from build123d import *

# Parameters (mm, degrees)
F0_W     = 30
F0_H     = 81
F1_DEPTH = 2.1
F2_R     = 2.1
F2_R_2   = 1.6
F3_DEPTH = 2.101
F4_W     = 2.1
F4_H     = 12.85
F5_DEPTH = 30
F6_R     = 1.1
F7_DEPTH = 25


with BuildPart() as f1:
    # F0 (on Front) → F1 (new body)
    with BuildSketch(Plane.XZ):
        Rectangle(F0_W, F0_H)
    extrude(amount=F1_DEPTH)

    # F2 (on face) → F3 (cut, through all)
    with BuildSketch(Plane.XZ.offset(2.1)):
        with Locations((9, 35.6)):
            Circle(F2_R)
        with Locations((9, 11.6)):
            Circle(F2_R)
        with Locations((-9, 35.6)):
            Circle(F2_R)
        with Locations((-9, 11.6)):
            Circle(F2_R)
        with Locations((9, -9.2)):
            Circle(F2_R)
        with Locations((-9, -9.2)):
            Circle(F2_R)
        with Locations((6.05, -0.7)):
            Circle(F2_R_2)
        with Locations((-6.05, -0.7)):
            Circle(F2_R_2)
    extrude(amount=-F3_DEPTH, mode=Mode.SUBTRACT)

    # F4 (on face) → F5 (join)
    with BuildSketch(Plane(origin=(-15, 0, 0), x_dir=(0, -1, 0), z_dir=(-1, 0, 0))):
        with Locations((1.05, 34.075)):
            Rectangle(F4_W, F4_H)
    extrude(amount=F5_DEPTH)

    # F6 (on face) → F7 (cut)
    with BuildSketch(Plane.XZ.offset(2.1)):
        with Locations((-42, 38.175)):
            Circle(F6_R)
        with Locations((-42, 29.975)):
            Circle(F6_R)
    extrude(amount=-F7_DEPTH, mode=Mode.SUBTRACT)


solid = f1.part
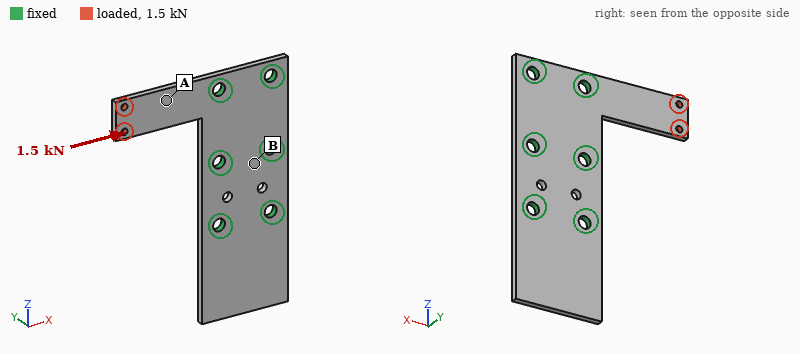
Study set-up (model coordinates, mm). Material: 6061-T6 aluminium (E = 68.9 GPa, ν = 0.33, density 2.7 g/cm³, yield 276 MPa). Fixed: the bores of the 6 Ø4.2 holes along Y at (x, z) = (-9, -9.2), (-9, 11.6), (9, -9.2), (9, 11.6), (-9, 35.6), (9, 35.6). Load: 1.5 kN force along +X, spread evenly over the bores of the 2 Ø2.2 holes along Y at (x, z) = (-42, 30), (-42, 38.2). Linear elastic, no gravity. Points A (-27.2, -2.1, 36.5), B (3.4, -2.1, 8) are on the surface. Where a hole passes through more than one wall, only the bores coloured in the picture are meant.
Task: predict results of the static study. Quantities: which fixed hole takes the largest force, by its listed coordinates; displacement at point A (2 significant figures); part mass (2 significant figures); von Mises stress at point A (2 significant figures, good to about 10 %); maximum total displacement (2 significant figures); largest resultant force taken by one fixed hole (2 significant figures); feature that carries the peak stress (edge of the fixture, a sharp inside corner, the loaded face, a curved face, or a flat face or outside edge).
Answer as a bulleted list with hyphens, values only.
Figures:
- (-9, 35.6)
- 15 µm
- 15 g
- 56 MPa
- 30 µm
- 1.3 kN
- the loaded face
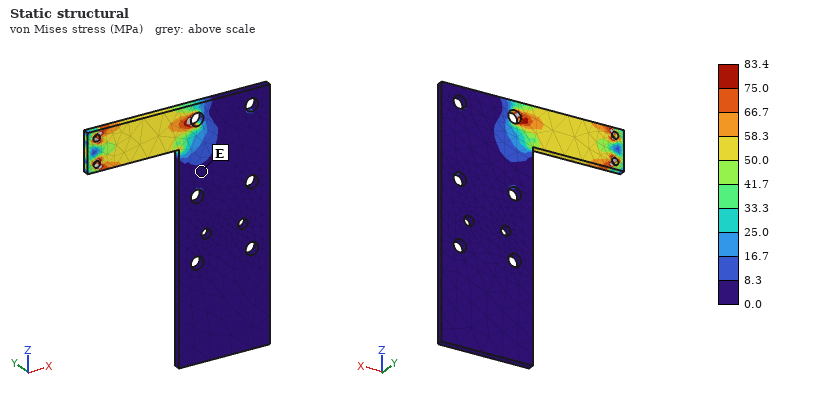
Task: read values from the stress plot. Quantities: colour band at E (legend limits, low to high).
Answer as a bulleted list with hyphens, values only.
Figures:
- 0.0 to 8.3 MPa
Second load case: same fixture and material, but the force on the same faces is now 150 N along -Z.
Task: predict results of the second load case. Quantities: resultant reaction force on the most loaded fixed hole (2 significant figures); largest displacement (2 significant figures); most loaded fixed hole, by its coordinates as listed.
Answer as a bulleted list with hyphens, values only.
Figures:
- 230 N
- 86 µm
- (-9, 35.6)
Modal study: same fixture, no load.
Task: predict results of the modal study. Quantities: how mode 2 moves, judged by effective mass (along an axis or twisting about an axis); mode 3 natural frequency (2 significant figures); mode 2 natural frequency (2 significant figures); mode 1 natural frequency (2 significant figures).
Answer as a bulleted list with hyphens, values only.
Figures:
- along Y
- 4600 Hz
- 1900 Hz
- 1500 Hz
